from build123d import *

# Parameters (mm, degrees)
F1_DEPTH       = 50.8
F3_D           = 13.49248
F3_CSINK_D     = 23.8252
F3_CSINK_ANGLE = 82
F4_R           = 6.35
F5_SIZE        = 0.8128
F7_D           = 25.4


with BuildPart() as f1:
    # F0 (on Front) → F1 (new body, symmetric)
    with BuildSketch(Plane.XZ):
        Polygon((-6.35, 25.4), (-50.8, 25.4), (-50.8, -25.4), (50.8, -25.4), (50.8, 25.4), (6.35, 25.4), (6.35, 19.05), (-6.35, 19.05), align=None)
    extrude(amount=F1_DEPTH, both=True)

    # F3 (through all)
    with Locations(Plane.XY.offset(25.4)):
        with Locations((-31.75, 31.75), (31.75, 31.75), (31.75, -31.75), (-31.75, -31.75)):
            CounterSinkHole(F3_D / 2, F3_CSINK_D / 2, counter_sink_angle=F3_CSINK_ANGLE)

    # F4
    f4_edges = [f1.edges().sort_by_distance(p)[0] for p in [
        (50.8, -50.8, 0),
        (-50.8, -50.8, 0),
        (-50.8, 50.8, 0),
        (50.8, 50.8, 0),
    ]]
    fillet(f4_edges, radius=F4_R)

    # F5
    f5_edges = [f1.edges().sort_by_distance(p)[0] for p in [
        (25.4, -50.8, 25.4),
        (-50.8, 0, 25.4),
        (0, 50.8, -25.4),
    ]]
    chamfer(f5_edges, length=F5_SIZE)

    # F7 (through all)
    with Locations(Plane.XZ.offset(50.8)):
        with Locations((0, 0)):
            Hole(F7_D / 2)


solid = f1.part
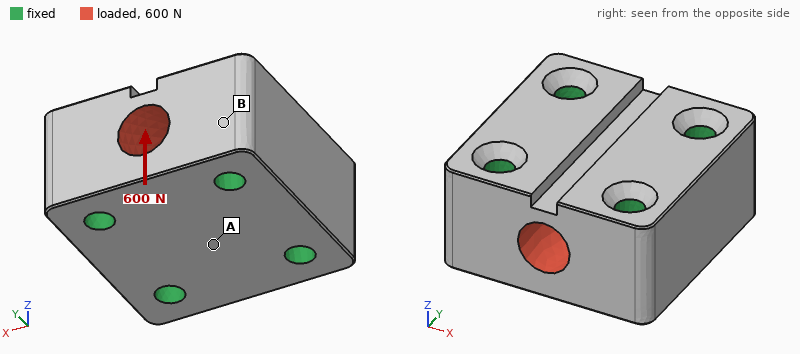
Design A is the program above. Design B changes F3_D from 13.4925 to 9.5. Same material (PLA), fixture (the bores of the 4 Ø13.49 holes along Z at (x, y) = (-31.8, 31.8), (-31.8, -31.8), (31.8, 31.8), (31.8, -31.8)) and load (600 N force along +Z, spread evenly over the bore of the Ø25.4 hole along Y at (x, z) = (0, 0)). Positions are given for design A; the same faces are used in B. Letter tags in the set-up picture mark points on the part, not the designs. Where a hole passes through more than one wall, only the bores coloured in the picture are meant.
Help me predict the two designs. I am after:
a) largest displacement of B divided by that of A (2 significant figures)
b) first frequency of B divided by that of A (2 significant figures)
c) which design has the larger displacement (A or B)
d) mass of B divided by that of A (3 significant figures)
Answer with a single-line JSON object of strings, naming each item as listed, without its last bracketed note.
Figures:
{"largest displacement of B divided by that of A": "1.1", "first frequency of B divided by that of A": "0.89", "which design has the larger displacement": "B", "mass of B divided by that of A": "1.03"}
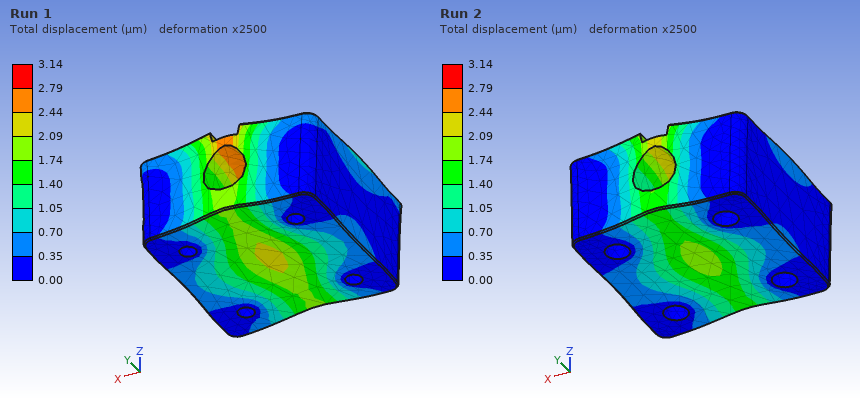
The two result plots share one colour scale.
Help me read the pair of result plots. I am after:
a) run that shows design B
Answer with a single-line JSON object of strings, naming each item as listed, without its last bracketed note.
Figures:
{"run that shows design B": "Run 1"}
